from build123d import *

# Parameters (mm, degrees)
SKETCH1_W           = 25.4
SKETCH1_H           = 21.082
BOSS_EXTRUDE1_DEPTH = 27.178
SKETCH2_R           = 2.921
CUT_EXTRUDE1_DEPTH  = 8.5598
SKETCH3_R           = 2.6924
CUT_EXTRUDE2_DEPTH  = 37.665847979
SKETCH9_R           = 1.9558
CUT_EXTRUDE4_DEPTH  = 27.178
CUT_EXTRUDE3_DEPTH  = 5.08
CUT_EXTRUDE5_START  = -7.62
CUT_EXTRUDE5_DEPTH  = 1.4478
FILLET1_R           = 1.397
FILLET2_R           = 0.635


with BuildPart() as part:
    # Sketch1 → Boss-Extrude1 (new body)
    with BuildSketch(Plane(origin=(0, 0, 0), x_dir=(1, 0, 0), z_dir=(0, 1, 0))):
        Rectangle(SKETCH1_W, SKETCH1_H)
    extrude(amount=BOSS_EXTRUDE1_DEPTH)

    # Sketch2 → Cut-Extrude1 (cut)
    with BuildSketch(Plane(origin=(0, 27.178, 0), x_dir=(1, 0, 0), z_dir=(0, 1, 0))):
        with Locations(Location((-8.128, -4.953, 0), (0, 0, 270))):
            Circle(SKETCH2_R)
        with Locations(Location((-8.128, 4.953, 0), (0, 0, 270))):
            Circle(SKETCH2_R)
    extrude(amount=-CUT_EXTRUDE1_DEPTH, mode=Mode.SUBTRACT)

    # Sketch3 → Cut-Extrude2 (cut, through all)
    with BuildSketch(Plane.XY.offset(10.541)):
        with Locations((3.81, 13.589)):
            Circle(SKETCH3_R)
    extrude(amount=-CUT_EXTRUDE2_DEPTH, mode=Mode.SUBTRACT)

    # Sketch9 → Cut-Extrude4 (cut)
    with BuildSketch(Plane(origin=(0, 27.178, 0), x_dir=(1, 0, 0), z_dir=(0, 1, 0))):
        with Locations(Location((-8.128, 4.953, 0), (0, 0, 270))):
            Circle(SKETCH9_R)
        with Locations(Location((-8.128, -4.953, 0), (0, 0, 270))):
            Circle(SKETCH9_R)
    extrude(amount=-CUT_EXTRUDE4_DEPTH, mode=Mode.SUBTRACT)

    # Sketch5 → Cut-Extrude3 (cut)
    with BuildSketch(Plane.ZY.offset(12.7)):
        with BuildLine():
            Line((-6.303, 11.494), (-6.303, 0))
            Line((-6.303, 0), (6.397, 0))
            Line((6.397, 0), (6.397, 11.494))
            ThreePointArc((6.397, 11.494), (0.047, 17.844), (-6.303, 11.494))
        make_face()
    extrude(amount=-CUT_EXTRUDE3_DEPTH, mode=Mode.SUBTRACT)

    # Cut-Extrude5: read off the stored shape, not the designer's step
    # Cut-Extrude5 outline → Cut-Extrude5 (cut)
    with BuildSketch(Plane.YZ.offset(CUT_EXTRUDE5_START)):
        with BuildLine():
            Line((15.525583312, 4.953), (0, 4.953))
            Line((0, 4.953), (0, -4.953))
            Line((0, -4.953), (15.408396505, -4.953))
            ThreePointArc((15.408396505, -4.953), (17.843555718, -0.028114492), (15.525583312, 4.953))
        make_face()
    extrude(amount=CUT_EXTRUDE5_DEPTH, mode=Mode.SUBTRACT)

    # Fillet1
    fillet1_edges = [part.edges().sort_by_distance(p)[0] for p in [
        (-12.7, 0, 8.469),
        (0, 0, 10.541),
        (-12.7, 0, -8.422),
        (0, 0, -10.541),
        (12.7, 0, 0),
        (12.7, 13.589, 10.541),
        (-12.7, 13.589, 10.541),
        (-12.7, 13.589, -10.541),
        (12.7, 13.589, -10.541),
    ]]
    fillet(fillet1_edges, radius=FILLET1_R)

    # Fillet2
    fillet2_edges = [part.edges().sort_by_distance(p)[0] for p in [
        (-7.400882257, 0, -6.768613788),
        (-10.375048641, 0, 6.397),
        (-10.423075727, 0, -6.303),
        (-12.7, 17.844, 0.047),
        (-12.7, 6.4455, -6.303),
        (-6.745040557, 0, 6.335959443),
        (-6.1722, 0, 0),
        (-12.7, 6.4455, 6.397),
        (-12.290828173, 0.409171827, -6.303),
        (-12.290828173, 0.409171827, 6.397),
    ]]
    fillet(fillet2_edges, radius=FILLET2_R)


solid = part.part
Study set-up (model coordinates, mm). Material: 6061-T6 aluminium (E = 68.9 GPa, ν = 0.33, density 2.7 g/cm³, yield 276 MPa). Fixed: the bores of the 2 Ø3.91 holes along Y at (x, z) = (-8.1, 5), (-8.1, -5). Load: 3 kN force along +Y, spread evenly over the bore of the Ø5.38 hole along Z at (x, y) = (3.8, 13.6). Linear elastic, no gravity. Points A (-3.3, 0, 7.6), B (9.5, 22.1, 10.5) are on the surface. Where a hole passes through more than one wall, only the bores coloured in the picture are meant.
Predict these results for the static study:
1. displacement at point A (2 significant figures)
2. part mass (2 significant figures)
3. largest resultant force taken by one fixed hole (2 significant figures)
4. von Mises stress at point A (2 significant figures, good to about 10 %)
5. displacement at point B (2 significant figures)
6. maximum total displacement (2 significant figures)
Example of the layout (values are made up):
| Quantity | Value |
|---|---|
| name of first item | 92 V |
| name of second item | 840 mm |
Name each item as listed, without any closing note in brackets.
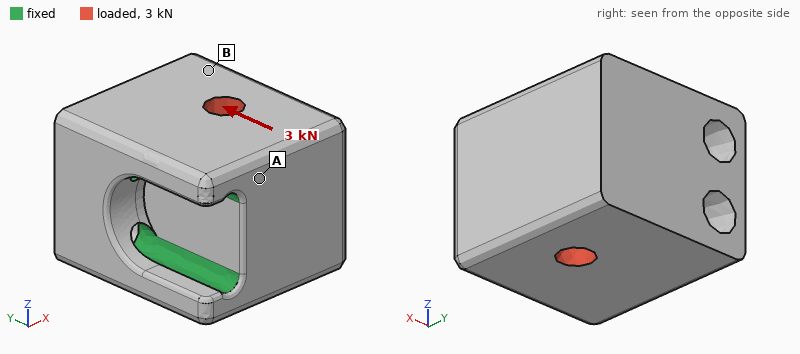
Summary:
| Quantity | Value |
|---|---|
| displacement at point A | 3.7 µm |
| part mass | 33 g |
| largest resultant force taken by one fixed hole | 1.5 kN |
| von Mises stress at point A | 20 MPa |
| displacement at point B | 10 µm |
| maximum total displacement | 13 µm |
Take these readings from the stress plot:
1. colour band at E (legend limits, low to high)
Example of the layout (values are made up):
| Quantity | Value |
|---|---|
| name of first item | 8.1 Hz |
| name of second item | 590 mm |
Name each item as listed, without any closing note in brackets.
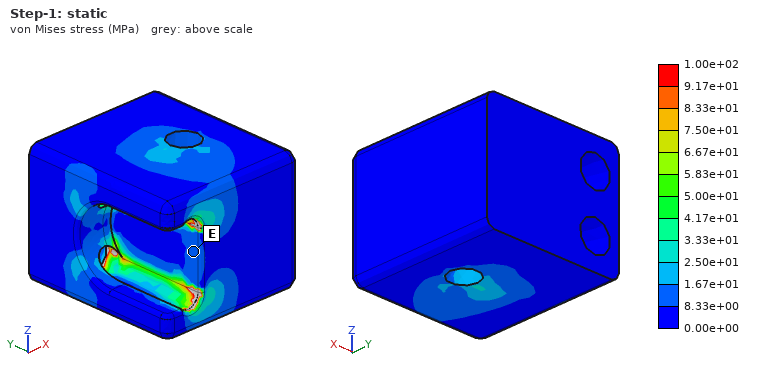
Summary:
| Quantity | Value |
|---|---|
| colour band at E | 8.33e+00 to 1.67e+01 MPa |
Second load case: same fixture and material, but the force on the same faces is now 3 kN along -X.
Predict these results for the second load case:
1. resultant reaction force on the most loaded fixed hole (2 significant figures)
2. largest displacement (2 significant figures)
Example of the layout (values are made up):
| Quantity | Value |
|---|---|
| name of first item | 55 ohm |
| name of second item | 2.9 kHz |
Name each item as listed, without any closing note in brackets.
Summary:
| Quantity | Value |
|---|---|
| resultant reaction force on the most loaded fixed hole | 1.5 kN |
| largest displacement | 3.3 µm |
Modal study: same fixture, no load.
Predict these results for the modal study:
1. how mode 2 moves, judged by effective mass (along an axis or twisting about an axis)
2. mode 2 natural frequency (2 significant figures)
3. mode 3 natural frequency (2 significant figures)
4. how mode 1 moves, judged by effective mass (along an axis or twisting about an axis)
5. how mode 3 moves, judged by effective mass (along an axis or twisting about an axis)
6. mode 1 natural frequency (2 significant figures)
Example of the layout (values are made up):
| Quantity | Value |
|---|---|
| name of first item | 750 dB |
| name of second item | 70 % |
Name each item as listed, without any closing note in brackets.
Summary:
| Quantity | Value |
|---|---|
| how mode 2 moves, judged by effective mass | along Z |
| mode 2 natural frequency | 19 kHz |
| mode 3 natural frequency | 28 kHz |
| how mode 1 moves, judged by effective mass | along Y |
| how mode 3 moves, judged by effective mass | twisting about X |
| mode 1 natural frequency | 17 kHz |
